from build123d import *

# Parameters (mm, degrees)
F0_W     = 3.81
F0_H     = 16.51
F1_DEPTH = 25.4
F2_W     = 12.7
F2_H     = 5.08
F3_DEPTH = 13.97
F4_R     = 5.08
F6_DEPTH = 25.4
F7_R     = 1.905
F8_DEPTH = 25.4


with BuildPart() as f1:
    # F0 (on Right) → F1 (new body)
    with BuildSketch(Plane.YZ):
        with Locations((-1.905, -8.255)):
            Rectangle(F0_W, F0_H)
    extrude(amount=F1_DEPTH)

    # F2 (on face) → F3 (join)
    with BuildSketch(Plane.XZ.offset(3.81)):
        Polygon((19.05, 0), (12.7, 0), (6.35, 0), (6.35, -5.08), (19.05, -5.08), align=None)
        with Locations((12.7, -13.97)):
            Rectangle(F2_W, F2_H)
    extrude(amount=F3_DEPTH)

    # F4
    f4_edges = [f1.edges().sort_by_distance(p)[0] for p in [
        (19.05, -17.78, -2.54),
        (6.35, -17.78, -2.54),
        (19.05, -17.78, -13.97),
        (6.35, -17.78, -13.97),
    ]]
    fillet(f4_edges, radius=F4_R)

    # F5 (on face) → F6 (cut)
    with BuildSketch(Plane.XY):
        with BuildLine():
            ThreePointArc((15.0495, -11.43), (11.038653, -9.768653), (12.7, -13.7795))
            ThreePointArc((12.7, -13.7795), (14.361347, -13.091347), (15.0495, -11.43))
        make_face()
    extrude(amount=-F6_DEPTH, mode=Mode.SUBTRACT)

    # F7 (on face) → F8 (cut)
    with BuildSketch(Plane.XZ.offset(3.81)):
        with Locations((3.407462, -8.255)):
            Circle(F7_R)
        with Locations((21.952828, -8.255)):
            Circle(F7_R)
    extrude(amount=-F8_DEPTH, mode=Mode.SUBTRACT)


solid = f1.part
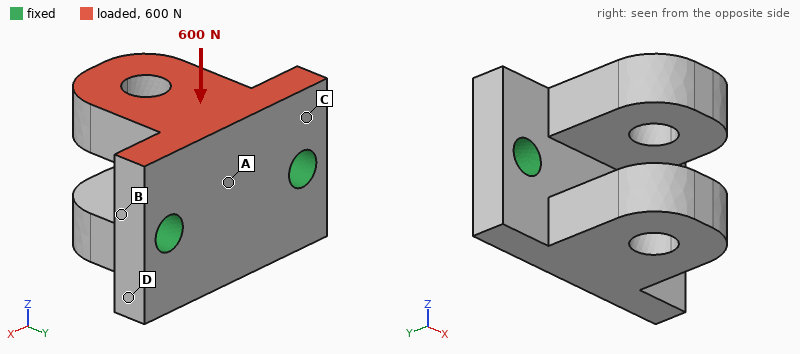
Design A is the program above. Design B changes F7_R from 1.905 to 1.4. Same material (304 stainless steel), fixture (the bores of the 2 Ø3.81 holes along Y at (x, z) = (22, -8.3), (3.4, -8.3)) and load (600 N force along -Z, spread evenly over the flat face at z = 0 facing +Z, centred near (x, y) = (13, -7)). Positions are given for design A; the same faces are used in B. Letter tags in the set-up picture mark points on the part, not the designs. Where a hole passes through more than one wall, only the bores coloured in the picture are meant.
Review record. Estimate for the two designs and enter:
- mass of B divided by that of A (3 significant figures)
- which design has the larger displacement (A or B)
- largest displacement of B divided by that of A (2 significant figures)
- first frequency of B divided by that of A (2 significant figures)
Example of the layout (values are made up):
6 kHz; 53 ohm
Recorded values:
1.01; B; 1.1; 0.92
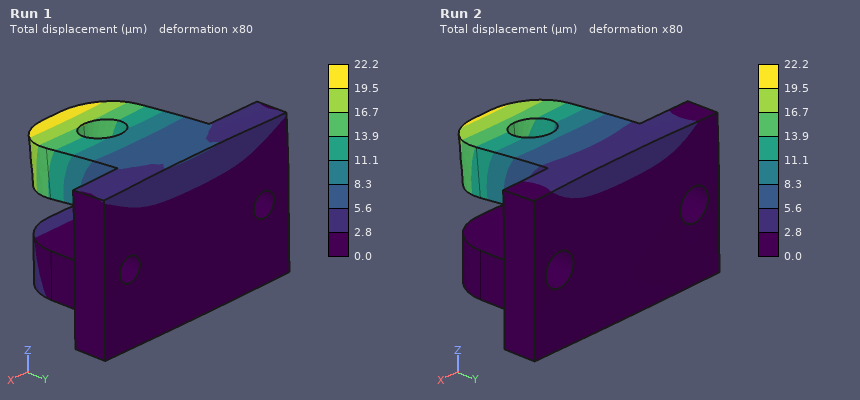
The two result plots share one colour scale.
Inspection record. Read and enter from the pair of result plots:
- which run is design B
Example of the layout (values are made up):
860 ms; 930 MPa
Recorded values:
Run 1
